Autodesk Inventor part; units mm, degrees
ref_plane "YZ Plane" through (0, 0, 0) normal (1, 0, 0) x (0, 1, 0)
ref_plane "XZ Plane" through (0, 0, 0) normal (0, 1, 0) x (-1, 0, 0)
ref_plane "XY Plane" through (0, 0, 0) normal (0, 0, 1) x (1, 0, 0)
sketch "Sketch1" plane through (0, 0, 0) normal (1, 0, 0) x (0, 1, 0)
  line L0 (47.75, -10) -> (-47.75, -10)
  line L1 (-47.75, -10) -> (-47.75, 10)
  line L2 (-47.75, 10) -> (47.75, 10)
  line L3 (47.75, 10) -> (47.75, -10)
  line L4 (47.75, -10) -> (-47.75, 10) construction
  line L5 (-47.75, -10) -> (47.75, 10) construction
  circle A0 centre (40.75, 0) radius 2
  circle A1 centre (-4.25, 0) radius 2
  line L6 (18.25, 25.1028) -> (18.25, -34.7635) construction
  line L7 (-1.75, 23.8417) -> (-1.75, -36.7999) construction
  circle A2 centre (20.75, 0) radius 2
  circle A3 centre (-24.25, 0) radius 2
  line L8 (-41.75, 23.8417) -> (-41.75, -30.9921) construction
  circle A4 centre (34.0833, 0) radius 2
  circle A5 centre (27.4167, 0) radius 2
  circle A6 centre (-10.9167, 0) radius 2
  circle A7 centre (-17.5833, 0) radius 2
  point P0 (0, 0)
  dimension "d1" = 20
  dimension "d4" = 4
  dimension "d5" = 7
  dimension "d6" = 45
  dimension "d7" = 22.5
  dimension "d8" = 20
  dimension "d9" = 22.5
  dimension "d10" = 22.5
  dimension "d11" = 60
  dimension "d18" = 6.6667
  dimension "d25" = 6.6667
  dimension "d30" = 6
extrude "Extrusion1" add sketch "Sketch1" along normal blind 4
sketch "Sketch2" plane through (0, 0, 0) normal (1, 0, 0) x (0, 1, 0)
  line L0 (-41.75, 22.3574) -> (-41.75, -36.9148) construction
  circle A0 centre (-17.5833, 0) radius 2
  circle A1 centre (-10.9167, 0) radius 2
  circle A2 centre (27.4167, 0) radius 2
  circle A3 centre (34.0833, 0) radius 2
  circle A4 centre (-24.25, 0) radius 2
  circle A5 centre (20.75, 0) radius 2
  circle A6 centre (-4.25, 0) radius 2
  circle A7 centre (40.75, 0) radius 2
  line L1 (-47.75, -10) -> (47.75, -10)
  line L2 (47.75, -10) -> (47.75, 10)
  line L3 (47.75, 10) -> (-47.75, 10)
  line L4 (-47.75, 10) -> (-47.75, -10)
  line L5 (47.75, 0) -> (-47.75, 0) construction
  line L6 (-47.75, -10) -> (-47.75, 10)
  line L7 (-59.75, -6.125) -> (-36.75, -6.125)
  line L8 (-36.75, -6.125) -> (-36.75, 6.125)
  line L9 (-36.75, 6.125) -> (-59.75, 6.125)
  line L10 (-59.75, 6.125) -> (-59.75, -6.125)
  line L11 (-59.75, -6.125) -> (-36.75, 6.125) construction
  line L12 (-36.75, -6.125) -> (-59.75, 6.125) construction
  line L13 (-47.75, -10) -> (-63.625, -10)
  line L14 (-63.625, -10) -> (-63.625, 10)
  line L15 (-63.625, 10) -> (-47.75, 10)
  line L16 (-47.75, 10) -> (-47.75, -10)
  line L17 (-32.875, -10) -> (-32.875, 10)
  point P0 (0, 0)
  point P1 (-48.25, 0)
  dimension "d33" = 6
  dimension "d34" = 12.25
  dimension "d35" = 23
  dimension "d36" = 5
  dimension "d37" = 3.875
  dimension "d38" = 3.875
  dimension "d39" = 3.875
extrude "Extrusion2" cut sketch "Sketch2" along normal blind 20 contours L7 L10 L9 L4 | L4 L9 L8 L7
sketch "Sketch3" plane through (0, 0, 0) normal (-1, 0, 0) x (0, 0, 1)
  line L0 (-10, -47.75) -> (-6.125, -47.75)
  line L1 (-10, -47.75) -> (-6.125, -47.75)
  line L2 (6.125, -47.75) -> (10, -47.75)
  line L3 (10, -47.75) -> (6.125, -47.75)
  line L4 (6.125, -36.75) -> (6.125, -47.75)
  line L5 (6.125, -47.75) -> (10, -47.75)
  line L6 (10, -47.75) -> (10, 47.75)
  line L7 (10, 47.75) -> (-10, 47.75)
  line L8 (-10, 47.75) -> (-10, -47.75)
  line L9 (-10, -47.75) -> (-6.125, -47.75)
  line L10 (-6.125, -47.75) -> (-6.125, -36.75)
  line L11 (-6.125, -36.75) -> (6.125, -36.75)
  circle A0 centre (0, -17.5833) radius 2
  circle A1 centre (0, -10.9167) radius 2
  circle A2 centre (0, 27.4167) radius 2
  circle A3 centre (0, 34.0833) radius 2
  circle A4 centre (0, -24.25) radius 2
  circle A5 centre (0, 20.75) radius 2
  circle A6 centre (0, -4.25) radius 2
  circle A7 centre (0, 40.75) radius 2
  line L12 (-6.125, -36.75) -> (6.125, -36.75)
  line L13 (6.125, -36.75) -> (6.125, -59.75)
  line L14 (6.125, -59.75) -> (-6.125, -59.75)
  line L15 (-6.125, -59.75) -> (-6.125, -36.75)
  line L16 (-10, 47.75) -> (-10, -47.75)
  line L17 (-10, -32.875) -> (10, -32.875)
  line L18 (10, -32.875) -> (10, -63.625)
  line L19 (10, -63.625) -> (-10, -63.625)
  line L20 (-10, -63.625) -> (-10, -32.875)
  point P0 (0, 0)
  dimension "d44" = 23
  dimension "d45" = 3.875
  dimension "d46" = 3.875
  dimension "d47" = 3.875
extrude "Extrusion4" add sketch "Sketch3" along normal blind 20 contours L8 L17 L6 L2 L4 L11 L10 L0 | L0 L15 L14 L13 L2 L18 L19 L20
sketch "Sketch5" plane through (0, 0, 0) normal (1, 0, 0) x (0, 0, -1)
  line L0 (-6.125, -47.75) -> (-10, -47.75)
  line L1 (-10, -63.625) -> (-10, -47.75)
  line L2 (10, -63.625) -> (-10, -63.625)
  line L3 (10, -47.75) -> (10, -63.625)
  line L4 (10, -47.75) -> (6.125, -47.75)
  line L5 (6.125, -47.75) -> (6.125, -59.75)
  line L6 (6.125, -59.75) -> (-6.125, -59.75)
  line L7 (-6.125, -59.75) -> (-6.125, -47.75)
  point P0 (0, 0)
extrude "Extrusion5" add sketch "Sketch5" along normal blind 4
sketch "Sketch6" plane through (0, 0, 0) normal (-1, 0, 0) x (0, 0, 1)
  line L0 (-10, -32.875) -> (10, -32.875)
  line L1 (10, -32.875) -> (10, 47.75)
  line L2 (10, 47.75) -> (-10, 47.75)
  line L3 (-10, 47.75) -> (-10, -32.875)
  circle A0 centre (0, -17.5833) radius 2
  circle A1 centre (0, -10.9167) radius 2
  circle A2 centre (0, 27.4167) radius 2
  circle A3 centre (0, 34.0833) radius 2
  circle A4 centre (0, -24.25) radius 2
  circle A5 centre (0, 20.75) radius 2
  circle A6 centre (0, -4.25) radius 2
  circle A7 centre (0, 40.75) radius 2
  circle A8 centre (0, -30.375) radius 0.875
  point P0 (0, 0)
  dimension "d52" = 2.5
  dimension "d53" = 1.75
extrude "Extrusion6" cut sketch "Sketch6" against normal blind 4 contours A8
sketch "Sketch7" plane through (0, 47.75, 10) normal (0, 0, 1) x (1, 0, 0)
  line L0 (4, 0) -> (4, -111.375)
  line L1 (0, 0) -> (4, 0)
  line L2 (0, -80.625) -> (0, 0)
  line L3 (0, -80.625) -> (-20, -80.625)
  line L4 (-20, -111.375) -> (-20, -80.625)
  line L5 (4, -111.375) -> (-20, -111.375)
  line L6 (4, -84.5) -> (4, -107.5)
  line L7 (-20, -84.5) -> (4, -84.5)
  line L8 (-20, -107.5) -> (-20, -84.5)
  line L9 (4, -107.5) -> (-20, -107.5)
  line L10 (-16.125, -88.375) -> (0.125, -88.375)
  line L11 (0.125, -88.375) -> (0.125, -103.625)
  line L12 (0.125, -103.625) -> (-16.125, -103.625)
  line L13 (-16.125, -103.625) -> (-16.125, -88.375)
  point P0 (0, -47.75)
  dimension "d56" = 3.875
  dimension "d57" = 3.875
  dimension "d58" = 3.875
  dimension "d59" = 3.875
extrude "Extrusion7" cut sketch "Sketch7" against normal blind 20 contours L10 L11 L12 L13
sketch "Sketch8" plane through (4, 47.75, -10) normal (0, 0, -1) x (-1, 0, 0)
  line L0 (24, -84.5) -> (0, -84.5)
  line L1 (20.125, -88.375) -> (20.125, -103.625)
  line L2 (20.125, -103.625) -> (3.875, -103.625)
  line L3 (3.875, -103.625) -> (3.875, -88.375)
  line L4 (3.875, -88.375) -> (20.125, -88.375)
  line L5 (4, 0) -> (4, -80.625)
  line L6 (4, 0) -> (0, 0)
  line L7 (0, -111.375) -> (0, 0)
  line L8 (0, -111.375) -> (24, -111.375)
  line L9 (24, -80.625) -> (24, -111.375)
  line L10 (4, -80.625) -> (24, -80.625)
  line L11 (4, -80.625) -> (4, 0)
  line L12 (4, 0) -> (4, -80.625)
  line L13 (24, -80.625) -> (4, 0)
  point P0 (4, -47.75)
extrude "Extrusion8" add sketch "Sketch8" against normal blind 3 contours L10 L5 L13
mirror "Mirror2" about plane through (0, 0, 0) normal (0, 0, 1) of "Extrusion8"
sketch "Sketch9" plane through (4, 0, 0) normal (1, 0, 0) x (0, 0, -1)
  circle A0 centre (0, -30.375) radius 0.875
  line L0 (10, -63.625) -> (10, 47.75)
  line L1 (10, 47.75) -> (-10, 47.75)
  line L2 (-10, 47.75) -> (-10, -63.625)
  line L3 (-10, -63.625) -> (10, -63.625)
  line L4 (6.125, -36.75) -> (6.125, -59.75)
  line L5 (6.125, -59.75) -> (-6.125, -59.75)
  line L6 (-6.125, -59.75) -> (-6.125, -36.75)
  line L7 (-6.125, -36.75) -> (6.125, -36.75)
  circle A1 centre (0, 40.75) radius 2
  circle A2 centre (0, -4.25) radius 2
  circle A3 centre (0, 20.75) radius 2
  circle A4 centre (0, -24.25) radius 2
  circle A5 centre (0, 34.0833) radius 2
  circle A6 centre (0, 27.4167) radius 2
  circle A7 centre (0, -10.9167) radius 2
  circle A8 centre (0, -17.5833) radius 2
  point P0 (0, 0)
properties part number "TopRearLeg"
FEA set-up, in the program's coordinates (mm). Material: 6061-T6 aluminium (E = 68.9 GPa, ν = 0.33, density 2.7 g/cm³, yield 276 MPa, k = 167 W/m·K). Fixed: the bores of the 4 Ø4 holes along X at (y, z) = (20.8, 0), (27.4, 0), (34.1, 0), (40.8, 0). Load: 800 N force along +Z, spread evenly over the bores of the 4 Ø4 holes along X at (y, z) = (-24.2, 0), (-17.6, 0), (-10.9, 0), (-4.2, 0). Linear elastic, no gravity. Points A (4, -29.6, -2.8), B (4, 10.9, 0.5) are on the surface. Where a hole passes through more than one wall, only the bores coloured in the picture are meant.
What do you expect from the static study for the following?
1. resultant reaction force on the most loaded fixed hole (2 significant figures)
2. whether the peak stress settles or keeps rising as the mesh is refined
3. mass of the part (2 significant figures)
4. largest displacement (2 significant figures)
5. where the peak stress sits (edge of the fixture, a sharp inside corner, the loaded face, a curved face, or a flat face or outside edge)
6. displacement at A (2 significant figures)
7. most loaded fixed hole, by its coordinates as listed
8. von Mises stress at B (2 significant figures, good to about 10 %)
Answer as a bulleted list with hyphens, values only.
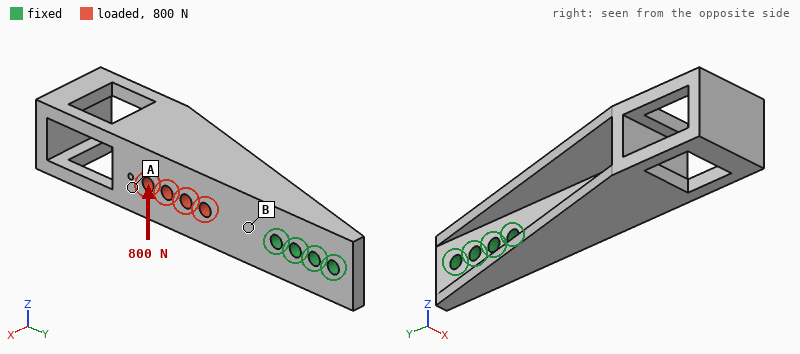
- 2.1 kN
- keeps rising
- 46 g
- 0.21 mm
- edge of the fixture
- 0.12 mm
- (20.8, 0)
- 25 MPa
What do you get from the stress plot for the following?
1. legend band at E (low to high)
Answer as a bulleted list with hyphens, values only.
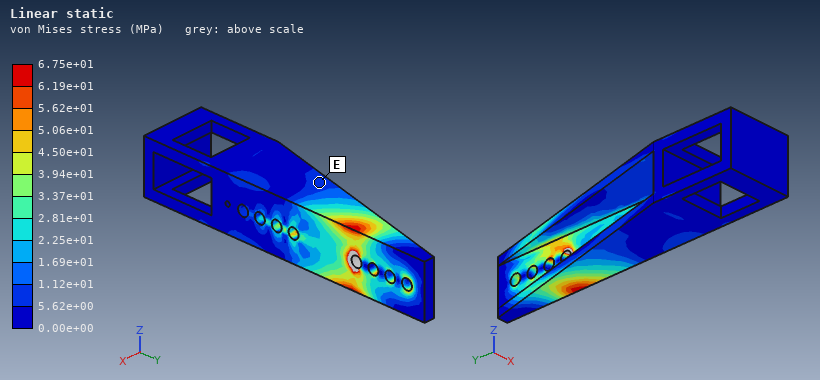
- 5.62e+00 to 1.12e+01 MPa
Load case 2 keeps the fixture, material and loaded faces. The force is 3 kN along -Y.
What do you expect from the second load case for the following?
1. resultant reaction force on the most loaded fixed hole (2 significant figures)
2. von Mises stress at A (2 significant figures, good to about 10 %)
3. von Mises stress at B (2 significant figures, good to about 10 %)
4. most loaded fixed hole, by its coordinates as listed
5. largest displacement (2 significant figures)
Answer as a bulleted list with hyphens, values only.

- 2.0 kN
- 7.4 MPa
- 49 MPa
- (20.8, 0)
- 0.13 mm
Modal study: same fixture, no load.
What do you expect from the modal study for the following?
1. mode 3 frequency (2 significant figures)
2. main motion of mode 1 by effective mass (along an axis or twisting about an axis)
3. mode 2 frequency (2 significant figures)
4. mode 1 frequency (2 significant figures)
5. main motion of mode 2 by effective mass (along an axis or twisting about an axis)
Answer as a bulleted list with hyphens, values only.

- 2300 Hz
- along X
- 1300 Hz
- 900 Hz
- along Z
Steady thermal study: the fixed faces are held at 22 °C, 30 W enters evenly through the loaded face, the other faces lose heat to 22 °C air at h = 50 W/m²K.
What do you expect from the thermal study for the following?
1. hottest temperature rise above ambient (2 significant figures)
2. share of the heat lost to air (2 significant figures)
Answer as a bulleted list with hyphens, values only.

- 35 K
- 37 %
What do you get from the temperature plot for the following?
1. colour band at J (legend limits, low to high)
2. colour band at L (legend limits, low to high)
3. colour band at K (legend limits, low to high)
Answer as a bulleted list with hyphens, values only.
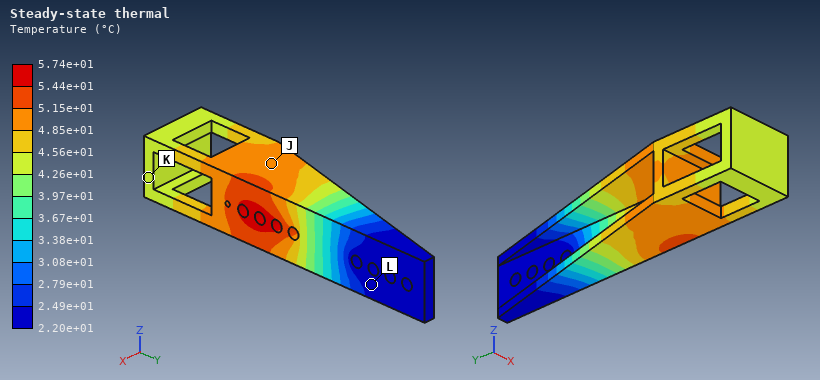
- 4.85e+01 to 5.15e+01 °C
- 2.20e+01 to 2.49e+01 °C
- 4.26e+01 to 4.56e+01 °C
